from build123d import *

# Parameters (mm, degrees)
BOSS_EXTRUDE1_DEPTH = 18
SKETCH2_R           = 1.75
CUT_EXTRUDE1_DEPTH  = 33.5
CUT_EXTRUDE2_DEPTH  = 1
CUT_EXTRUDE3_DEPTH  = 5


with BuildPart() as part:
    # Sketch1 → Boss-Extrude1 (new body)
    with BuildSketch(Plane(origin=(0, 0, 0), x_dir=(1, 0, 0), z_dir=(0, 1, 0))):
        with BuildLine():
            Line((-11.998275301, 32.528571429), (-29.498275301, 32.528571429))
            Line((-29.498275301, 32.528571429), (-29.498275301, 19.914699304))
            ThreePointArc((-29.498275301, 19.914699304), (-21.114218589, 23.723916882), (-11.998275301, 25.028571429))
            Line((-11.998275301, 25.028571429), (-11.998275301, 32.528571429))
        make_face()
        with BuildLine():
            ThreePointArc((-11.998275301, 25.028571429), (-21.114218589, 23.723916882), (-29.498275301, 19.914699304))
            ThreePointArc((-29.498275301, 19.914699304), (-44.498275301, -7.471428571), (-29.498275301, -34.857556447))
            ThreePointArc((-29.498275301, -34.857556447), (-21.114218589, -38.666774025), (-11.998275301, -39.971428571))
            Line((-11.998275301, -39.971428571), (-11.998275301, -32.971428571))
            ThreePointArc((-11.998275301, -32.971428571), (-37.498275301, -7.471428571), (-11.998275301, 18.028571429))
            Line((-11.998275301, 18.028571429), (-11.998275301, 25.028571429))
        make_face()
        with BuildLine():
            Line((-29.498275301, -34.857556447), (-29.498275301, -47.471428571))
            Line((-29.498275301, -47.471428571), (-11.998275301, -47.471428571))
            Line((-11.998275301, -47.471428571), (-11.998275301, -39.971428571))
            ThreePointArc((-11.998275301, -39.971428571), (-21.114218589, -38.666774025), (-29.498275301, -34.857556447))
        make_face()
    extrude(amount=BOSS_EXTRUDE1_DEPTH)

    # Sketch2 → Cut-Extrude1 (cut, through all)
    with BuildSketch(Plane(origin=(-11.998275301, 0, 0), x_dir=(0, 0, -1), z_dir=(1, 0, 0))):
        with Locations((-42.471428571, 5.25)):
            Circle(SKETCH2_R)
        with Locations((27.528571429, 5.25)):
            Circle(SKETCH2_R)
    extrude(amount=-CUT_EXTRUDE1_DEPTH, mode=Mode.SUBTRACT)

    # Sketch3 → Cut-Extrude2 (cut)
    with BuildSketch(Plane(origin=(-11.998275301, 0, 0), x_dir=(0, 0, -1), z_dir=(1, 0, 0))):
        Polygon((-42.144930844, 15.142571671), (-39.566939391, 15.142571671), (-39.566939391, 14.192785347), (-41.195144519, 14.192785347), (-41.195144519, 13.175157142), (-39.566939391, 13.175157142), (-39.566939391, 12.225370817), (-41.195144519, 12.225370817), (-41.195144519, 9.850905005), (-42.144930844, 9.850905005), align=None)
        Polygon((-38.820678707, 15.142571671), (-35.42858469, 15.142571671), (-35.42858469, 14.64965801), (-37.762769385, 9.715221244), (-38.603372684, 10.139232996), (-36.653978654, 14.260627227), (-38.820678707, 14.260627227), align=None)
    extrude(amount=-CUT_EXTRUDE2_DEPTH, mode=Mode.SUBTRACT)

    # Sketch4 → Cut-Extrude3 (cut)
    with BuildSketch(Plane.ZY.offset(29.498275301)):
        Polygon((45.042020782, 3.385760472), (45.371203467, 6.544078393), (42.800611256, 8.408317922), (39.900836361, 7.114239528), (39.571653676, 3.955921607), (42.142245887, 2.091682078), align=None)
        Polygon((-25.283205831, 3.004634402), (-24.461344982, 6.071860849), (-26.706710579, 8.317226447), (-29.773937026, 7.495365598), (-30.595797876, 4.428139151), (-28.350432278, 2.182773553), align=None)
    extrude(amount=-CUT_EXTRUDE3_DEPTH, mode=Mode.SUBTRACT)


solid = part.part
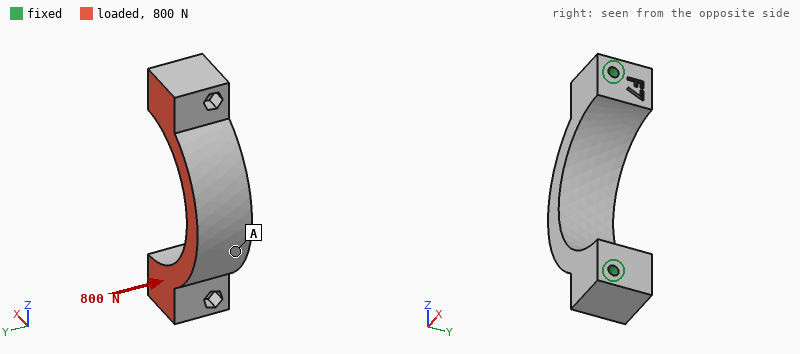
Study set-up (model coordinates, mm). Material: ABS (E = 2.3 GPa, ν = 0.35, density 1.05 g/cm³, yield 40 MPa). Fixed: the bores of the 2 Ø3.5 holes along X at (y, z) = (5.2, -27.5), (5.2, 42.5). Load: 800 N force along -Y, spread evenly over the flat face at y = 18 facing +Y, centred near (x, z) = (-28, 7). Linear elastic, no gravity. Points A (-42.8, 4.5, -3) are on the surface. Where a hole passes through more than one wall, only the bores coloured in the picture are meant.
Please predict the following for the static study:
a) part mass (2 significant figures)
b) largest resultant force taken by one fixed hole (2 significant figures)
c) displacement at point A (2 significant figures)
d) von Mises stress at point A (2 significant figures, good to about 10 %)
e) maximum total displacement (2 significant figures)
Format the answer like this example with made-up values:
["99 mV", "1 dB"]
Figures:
["18 g", "400 N", "0.38 mm", "3.6 MPa", "0.47 mm"]
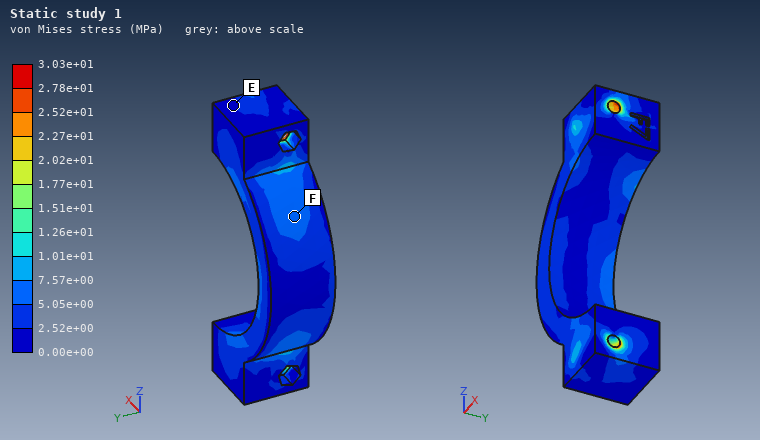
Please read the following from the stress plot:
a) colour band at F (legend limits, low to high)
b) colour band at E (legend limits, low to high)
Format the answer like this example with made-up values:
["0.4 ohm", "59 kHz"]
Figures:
["5.05e+00 to 7.57e+00 MPa", "0.00e+00 to 2.52e+00 MPa"]
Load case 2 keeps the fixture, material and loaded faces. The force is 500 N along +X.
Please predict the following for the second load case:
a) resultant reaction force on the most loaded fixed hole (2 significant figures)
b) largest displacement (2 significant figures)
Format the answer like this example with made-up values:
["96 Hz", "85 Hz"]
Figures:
["260 N", "0.24 mm"]
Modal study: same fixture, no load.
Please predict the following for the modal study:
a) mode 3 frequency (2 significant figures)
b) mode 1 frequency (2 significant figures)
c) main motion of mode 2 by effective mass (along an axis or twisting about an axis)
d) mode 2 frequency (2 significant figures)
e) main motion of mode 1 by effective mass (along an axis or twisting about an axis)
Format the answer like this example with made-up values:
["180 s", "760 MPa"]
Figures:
["5000 Hz", "1900 Hz", "along Z", "3700 Hz", "along Y"]
